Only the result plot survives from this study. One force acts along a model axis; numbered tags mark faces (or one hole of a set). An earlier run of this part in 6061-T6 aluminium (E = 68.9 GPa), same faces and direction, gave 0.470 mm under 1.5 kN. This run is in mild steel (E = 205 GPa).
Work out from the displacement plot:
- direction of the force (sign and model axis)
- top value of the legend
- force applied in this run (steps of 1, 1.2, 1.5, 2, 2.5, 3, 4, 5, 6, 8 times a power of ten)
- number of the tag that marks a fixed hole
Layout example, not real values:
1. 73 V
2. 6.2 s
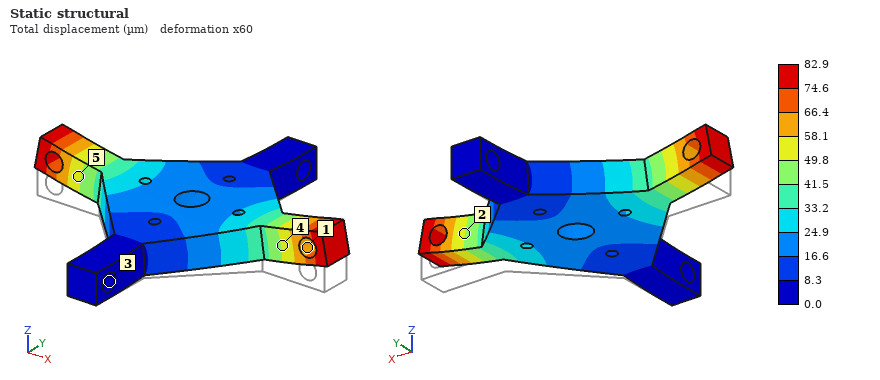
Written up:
1. +Z
2. 82.9 µm
3. 800 N
4. 3
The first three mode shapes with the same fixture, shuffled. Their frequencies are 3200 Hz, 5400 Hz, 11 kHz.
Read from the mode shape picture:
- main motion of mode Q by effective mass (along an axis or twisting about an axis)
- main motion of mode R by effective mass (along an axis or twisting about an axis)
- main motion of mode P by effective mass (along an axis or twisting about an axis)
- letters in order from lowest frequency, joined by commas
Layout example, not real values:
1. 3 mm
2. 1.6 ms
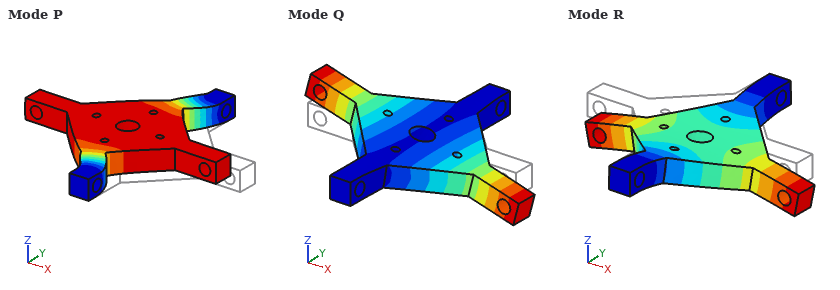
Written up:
1. twisting about Y
2. along Z
3. along X
4. Q, R, P
